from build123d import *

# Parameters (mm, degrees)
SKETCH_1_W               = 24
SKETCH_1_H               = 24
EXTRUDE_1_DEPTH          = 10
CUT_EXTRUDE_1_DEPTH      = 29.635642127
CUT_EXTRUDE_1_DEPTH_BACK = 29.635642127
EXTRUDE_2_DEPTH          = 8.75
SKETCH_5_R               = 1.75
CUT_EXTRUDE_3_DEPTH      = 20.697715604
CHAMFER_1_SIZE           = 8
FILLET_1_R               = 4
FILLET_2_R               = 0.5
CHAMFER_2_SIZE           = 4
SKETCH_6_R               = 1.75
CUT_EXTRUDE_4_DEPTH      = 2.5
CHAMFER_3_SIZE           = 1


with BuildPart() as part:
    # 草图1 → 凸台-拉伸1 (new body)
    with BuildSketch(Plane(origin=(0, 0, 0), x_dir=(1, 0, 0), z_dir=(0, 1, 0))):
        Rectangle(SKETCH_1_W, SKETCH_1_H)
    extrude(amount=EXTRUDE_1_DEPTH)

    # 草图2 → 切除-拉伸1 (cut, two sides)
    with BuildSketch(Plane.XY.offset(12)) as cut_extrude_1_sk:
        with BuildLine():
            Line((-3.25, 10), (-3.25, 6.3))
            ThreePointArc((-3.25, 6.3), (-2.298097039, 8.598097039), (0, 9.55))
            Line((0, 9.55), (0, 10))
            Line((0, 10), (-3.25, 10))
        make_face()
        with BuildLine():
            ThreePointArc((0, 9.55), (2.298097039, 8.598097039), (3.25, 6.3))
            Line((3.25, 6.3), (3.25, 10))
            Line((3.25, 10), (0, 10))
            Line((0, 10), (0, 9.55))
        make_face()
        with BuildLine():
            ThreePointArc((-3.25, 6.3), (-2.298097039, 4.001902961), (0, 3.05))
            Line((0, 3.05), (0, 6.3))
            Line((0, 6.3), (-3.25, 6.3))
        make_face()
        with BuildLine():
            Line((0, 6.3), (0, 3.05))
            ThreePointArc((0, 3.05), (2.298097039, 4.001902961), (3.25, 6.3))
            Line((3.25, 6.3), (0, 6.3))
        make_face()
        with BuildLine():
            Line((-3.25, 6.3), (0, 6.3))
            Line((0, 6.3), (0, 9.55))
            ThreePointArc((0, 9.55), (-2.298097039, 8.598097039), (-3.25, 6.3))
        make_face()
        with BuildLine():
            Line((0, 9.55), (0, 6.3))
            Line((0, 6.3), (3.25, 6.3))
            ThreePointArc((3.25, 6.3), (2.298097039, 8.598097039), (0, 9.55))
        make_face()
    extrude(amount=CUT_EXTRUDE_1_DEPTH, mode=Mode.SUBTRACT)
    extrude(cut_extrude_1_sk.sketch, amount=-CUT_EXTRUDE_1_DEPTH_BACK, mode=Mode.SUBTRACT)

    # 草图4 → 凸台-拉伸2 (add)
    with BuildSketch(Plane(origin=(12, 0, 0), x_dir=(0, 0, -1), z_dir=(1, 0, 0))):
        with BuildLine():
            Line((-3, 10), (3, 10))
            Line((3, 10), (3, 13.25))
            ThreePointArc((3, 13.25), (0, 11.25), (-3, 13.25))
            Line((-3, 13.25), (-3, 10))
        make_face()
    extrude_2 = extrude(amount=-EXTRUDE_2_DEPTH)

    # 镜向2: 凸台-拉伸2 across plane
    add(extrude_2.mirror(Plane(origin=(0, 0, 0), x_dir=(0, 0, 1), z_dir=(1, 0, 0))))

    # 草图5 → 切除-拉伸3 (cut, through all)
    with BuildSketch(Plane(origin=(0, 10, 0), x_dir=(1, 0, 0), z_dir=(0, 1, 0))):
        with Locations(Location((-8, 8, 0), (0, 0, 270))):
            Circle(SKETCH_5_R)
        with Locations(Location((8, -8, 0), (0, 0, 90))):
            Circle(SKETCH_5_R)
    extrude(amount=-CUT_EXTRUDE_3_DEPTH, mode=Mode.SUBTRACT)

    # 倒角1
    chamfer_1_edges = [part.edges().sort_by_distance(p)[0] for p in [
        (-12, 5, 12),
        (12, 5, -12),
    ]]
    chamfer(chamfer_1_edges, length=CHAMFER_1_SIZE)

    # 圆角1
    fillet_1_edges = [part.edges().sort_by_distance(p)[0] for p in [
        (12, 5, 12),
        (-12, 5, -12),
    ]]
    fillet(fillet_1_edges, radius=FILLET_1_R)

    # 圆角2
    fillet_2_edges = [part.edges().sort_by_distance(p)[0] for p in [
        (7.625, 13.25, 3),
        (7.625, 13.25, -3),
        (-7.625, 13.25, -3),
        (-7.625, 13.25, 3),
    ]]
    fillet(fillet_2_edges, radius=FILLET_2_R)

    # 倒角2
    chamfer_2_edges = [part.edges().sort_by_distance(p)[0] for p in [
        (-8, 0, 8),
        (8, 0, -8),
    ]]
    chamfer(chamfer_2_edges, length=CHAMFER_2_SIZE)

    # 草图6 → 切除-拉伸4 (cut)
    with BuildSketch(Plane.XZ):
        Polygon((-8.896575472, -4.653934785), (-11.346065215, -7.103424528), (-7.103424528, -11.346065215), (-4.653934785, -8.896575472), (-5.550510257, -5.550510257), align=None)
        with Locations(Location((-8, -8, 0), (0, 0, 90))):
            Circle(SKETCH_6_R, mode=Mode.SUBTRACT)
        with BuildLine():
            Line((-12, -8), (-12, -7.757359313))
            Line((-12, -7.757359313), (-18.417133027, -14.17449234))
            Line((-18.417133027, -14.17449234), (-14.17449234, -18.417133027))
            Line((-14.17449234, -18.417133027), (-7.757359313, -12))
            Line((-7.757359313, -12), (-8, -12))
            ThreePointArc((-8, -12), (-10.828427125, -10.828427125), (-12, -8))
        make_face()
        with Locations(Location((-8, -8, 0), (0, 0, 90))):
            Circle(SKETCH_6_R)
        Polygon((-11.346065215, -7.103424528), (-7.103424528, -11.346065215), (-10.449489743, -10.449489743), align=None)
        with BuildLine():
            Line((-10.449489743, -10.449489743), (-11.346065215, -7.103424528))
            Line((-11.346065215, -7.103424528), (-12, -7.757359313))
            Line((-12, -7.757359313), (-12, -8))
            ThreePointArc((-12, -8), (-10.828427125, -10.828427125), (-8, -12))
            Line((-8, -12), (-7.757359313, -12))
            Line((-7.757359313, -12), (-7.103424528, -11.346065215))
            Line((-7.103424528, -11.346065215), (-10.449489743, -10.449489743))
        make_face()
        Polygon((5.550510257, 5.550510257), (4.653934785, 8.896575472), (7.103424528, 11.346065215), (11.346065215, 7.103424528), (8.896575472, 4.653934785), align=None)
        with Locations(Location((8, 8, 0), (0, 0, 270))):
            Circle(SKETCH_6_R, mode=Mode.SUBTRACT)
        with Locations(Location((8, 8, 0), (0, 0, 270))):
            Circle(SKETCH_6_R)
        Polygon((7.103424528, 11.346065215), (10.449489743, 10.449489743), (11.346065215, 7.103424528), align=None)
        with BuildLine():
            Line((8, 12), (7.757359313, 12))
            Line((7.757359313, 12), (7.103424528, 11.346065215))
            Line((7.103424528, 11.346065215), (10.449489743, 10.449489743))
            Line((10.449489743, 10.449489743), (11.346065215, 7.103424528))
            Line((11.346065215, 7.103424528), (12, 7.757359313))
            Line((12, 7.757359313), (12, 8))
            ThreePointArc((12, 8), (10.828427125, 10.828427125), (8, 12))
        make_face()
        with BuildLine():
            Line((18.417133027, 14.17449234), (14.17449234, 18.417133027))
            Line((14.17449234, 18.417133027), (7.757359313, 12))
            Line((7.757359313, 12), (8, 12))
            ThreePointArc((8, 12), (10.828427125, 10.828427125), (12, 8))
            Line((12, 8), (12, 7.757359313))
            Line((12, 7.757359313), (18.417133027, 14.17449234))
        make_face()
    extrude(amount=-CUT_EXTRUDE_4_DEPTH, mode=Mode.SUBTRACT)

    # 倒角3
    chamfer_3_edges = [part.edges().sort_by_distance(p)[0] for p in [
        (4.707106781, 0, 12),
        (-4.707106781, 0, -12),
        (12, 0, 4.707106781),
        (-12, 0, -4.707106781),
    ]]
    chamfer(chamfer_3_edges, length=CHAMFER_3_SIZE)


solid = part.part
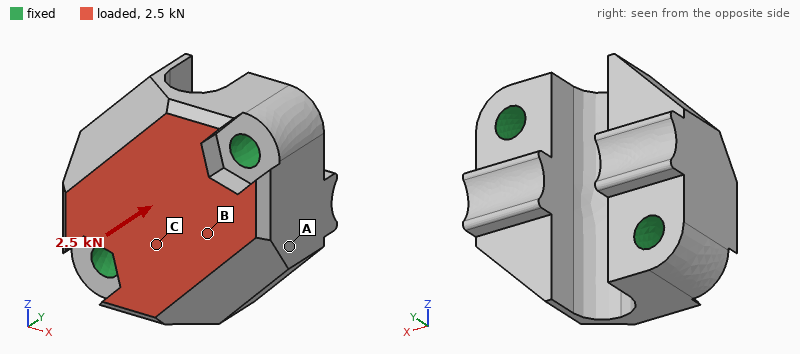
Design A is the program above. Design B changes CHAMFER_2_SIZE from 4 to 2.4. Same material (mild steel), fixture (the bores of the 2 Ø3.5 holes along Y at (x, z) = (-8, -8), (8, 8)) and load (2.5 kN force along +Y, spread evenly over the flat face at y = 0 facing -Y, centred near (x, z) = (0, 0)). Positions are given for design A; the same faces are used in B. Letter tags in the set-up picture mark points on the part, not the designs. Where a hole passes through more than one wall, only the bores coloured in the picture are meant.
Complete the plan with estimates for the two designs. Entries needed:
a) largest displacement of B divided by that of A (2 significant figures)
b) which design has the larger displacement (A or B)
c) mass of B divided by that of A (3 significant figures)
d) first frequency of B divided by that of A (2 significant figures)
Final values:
1.1
B
1.04
0.95
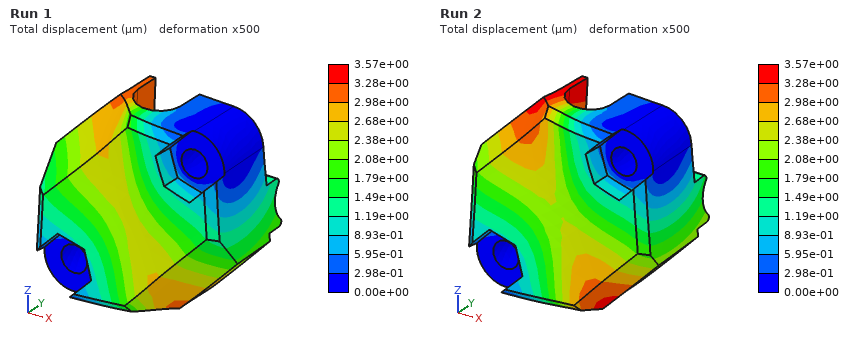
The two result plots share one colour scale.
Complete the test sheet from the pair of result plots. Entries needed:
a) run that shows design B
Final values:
Run 2
